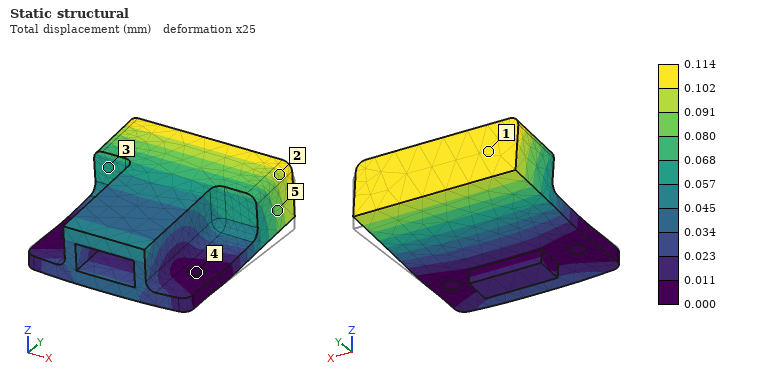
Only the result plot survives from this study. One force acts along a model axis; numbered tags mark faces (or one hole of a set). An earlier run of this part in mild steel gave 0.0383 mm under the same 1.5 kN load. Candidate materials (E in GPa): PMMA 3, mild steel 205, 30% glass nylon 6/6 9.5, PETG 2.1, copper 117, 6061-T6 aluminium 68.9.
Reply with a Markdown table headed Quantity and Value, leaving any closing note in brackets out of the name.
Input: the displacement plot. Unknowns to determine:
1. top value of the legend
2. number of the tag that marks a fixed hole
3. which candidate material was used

| Quantity | Value |
|---|---|
| top value of the legend | 0.114 mm |
| number of the tag that marks a fixed hole | 4 |
| which candidate material was used | 6061-T6 aluminium |
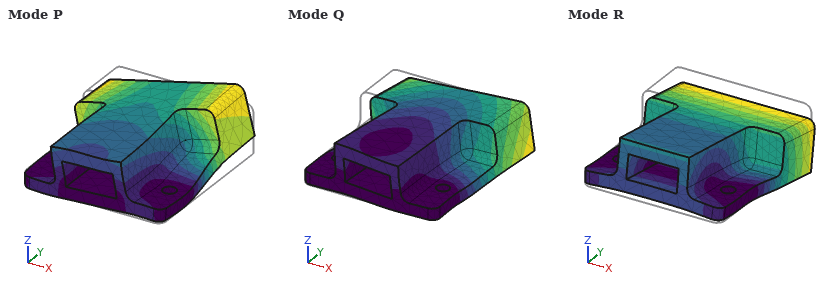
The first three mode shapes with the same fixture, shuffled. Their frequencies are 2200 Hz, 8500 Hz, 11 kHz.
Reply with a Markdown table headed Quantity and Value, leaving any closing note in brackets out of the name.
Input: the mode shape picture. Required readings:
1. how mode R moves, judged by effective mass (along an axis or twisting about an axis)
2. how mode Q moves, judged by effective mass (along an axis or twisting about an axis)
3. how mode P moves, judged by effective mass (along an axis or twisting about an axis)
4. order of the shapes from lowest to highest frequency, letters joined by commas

| Quantity | Value |
|---|---|
| how mode R moves, judged by effective mass | along Z |
| how mode Q moves, judged by effective mass | along X |
| how mode P moves, judged by effective mass | along X |
| order of the shapes from lowest to highest frequency, letters joined by commas | R, P, Q |
